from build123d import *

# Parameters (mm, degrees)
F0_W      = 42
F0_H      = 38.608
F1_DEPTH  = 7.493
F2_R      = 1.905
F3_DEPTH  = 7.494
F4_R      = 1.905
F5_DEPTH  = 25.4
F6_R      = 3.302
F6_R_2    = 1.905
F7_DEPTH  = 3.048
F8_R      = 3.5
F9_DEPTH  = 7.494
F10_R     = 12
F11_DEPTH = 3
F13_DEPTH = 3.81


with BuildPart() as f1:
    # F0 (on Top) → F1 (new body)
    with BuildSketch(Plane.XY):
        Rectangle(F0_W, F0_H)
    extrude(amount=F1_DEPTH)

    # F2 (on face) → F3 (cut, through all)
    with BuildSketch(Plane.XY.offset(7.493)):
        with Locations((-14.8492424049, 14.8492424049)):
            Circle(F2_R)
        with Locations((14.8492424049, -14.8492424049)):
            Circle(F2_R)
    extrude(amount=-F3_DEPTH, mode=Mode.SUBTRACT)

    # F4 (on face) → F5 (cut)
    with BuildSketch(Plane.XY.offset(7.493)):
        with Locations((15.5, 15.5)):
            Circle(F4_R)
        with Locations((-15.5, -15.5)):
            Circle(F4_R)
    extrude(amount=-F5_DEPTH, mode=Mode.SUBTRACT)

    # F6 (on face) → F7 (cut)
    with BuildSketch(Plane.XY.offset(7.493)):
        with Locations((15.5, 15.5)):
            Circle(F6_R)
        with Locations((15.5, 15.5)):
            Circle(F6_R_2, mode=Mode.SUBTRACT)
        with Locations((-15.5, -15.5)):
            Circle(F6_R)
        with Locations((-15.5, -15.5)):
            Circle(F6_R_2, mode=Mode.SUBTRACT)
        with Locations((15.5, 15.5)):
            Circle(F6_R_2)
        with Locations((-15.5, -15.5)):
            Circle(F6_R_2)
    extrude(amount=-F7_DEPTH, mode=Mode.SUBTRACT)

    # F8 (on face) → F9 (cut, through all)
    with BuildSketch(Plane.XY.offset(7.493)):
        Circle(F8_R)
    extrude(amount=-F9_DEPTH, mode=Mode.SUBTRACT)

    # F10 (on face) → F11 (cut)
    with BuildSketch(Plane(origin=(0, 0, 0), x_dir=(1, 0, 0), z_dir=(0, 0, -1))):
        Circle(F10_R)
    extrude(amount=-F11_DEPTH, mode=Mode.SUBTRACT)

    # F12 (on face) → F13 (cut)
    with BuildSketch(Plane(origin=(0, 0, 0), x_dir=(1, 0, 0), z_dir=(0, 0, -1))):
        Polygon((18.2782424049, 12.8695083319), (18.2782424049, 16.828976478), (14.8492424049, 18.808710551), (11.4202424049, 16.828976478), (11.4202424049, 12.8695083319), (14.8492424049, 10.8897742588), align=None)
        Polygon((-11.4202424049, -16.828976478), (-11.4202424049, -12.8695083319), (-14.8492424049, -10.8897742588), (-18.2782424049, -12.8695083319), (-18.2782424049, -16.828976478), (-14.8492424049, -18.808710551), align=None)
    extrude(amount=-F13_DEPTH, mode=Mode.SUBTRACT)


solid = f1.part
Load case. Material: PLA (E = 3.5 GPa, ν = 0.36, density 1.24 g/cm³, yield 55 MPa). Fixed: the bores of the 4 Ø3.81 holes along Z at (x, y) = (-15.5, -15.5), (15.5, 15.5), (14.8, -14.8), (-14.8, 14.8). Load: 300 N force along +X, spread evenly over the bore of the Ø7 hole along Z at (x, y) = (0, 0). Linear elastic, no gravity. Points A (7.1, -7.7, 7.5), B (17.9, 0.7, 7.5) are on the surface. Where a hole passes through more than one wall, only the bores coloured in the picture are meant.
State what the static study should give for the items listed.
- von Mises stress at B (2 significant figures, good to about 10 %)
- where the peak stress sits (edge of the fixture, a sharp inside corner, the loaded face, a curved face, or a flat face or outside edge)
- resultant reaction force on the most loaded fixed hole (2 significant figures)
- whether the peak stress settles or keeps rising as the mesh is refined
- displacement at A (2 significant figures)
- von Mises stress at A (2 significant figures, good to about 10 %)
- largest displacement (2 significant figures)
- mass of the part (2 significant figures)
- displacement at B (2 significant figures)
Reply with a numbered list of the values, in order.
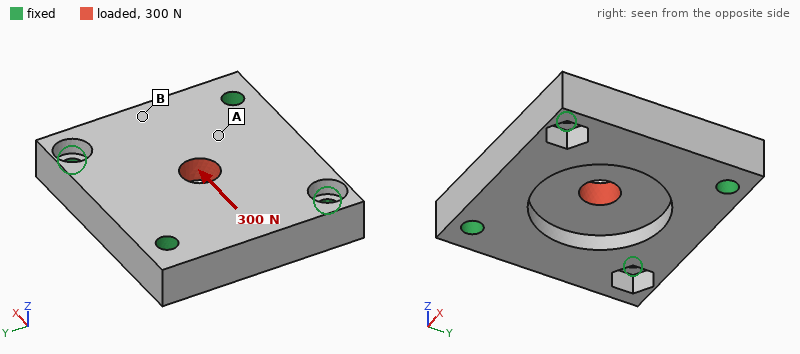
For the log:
1. 0.63 MPa
2. edge of the fixture
3. 82 N
4. keeps rising
5. 6.0 µm
6. 1.8 MPa
7. 13 µm
8. 12 g
9. 8.2 µm
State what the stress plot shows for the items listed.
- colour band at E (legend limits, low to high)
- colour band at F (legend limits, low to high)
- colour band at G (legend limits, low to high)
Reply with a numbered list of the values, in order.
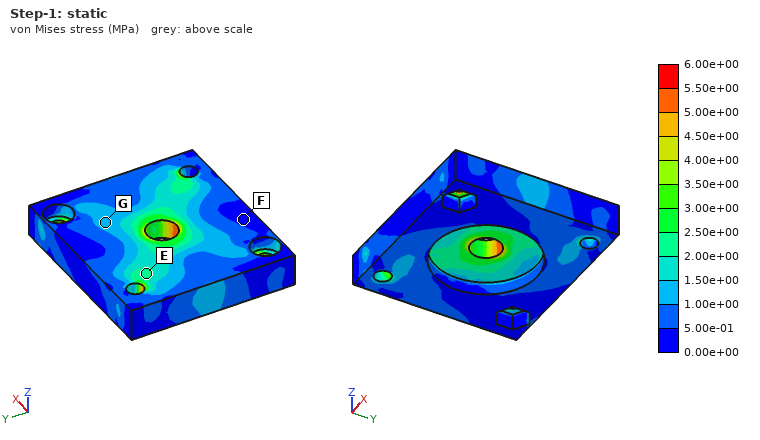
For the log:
1. 2.00e+00 to 2.50e+00 MPa
2. 0.00e+00 to 5.00e-01 MPa
3. 1.00e+00 to 1.50e+00 MPa
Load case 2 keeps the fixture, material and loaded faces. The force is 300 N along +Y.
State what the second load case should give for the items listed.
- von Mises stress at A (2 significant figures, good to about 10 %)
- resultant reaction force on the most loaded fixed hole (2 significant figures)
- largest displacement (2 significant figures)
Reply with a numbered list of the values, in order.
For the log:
1. 1.9 MPa
2. 84 N
3. 14 µm
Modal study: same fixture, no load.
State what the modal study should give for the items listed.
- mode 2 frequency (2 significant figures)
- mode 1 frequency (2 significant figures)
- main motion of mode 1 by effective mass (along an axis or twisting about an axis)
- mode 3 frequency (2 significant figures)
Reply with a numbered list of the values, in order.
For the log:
1. 8300 Hz
2. 6500 Hz
3. along Z
4. 8400 Hz
